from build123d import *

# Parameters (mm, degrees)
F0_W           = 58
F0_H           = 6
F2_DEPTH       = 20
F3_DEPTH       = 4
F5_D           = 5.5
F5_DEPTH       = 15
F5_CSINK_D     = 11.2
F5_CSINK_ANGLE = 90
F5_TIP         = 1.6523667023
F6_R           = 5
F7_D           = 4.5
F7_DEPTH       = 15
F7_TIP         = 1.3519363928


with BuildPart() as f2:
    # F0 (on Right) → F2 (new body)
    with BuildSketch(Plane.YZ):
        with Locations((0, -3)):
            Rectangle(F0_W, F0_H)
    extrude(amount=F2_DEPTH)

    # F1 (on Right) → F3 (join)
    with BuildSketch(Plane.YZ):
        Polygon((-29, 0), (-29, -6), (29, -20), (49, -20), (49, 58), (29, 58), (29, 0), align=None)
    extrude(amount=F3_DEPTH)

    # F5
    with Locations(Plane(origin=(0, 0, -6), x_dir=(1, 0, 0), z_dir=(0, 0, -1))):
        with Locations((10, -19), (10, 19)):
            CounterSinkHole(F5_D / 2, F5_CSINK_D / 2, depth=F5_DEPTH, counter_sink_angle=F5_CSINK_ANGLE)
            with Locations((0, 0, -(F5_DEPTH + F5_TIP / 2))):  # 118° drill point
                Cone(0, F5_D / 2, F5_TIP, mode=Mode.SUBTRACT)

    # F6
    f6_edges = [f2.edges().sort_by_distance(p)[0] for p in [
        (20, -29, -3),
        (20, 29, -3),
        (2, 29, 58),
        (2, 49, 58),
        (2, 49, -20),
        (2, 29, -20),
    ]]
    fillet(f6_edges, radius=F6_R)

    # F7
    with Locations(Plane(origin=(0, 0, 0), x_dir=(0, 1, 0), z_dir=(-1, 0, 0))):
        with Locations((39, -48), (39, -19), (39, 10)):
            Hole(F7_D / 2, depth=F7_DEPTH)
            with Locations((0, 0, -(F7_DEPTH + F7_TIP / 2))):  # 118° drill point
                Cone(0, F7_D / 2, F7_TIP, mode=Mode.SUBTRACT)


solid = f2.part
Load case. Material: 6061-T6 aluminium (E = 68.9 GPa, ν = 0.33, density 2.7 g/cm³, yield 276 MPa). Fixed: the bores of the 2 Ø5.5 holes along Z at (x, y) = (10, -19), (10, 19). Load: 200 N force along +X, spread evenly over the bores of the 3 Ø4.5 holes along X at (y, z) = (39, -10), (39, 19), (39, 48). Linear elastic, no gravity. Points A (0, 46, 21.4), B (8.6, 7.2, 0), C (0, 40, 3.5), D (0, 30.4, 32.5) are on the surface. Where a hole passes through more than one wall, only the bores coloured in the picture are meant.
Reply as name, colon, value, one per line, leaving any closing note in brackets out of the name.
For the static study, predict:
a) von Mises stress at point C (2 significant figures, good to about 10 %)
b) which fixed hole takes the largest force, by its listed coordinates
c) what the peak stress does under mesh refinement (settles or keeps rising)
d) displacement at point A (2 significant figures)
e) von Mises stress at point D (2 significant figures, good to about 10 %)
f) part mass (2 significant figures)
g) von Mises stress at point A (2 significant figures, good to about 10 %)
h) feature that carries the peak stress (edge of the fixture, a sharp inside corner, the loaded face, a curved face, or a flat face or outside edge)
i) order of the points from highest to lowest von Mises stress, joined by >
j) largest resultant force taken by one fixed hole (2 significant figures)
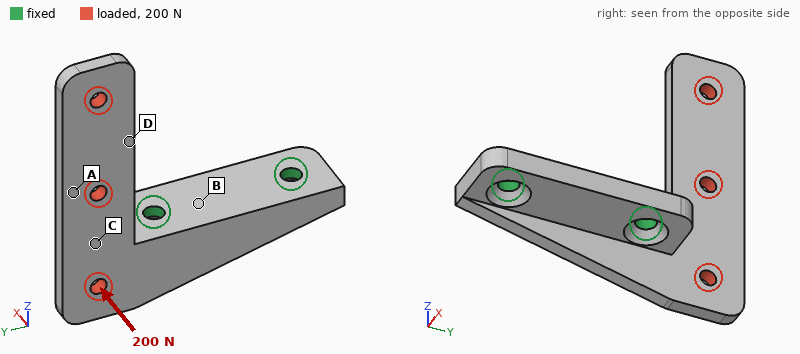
von Mises stress at point C: 70 MPa
which fixed hole takes the largest force, by its listed coordinates: (10, 19)
what the peak stress does under mesh refinement: keeps rising
displacement at point A: 0.38 mm
von Mises stress at point D: 20 MPa
part mass: 38 g
von Mises stress at point A: 39 MPa
feature that carries the peak stress: a sharp inside corner
order of the points from highest to lowest von Mises stress, joined by >: C > A > D > B
largest resultant force taken by one fixed hole: 280 N
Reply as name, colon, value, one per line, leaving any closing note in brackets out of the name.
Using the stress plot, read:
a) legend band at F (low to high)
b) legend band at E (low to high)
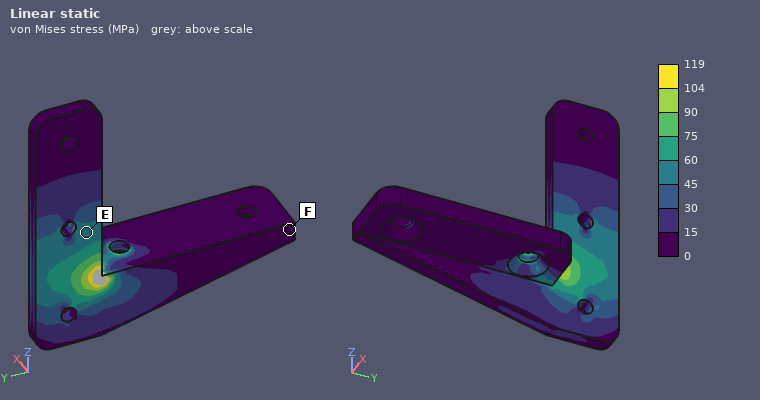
legend band at F: 0 to 15 MPa
legend band at E: 45 to 60 MPa
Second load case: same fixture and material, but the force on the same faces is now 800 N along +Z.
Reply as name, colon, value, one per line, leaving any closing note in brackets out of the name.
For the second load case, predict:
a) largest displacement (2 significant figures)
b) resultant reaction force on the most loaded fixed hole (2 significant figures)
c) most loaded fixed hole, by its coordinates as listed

largest displacement: 0.26 mm
resultant reaction force on the most loaded fixed hole: 1.3 kN
most loaded fixed hole, by its coordinates as listed: (10, 19)
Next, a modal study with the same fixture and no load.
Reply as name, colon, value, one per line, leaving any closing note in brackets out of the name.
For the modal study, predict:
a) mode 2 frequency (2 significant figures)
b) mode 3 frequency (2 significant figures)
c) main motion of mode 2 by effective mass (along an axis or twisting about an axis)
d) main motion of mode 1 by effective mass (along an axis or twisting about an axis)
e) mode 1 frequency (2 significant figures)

mode 2 frequency: 2000 Hz
mode 3 frequency: 3100 Hz
main motion of mode 2 by effective mass: along Y
main motion of mode 1 by effective mass: along X
mode 1 frequency: 670 Hz
